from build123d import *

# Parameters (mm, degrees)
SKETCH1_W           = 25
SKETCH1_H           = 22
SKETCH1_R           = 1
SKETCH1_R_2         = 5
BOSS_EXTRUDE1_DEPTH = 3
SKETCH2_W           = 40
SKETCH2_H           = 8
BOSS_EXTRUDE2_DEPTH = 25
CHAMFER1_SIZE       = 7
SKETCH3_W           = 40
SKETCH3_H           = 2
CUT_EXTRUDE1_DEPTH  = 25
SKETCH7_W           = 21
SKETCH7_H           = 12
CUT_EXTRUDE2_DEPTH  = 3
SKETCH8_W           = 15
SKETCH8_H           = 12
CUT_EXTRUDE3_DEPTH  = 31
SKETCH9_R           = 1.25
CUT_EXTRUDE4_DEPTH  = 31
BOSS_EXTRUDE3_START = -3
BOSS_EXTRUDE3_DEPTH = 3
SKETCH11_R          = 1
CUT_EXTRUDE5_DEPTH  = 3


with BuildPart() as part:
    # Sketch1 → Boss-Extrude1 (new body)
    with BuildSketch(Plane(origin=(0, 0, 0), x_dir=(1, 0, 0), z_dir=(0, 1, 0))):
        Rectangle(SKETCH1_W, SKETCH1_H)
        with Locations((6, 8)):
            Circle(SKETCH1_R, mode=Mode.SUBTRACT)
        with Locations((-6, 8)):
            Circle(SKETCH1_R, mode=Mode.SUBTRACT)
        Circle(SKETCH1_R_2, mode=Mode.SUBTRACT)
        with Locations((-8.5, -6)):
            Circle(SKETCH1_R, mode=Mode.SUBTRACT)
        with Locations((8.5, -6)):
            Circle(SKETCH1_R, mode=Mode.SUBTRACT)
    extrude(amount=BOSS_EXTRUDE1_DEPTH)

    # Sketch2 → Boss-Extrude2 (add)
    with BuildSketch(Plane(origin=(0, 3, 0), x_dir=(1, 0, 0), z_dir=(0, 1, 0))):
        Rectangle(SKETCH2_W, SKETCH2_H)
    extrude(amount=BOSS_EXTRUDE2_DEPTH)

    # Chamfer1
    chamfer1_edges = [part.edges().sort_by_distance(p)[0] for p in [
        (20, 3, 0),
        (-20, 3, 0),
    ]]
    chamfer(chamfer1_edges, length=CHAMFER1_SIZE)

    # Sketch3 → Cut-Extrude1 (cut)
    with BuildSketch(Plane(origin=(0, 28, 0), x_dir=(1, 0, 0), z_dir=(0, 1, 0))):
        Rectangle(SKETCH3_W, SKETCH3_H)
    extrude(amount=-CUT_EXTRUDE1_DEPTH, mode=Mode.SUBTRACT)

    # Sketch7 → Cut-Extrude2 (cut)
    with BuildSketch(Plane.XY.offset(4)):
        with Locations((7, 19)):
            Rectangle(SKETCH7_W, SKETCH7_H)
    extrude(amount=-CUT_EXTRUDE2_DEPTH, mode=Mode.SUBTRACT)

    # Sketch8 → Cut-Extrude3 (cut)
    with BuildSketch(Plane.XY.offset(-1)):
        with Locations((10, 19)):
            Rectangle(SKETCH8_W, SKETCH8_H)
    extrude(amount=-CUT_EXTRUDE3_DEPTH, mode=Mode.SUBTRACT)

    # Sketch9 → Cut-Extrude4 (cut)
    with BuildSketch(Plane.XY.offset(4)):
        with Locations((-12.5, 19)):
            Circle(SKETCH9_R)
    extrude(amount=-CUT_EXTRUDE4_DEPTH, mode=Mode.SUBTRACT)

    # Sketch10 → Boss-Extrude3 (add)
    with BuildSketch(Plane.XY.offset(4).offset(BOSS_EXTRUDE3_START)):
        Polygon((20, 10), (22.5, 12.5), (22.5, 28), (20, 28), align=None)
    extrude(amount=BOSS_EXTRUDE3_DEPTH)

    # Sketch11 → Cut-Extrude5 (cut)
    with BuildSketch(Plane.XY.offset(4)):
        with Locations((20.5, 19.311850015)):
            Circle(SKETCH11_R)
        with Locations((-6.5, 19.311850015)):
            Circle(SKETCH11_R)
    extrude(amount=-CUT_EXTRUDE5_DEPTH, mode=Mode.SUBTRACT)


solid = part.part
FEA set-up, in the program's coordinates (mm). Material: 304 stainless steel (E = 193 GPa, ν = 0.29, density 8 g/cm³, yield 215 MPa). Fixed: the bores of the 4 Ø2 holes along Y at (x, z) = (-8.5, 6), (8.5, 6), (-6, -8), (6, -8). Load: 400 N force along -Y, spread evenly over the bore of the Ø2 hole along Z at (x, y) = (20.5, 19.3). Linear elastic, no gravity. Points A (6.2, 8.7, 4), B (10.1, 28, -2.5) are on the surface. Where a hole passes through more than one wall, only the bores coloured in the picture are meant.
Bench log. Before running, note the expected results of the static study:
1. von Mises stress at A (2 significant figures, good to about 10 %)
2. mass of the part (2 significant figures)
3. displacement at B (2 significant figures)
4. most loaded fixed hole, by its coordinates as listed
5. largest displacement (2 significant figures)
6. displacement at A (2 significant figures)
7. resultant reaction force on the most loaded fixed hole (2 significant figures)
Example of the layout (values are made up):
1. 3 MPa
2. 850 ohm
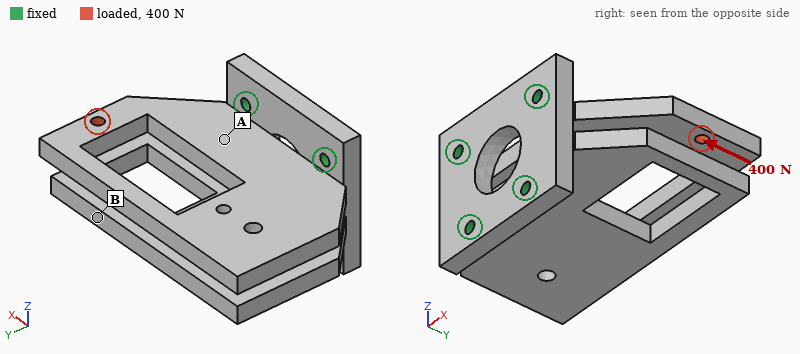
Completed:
1. 17 MPa
2. 47 g
3. 4.9 µm
4. (8.5, 6)
5. 15 µm
6. 2.7 µm
7. 540 N
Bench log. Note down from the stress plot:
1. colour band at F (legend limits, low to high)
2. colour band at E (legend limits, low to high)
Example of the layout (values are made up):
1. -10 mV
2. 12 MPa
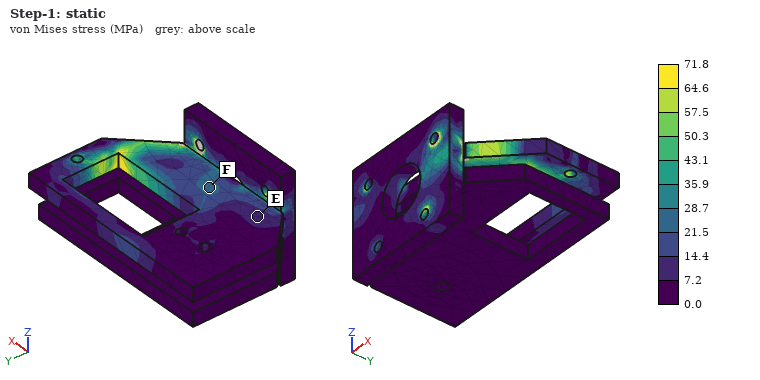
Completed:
1. 21.5 to 28.7 MPa
2. 7.2 to 14.4 MPa
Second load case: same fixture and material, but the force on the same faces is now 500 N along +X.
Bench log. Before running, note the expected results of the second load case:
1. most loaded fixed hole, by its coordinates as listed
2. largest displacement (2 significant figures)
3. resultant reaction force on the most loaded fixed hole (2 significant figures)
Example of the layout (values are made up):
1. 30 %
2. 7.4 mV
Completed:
1. (8.5, 6)
2. 21 µm
3. 480 N
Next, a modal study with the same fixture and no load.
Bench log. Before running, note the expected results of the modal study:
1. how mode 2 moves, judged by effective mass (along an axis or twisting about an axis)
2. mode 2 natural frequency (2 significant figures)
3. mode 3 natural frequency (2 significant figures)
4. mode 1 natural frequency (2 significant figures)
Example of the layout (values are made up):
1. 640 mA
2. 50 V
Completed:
1. along Z
2. 2800 Hz
3. 3900 Hz
4. 2600 Hz
